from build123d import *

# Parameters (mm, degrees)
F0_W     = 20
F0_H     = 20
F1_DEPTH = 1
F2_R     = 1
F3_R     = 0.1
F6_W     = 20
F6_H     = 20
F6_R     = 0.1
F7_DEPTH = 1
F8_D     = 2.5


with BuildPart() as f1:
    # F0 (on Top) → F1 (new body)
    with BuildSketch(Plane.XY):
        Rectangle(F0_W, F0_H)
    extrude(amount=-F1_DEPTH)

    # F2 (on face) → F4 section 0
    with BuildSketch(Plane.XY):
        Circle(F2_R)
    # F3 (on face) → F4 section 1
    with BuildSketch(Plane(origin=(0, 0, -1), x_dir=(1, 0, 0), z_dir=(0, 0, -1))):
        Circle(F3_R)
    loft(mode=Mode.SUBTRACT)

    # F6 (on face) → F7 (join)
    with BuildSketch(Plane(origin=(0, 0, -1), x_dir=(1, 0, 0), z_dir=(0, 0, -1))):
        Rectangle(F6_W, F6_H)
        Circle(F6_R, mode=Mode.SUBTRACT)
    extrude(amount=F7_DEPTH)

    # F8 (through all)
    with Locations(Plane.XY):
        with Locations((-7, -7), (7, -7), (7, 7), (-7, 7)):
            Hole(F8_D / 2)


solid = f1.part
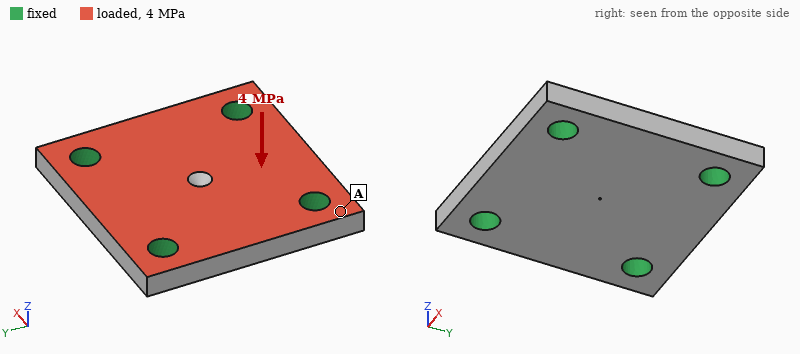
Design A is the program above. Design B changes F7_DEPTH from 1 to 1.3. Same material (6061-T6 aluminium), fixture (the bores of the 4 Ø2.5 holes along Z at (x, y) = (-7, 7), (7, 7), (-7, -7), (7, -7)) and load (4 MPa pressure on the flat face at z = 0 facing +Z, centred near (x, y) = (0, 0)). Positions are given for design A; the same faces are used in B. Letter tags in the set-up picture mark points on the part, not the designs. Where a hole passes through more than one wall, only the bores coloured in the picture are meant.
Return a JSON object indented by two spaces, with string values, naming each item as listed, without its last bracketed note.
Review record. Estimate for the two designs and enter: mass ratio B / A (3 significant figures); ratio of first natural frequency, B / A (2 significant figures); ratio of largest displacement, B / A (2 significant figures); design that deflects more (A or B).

{
  "mass ratio B / A": "1.15",
  "ratio of first natural frequency, B / A": "1.1",
  "ratio of largest displacement, B / A": "0.71",
  "design that deflects more": "A"
}
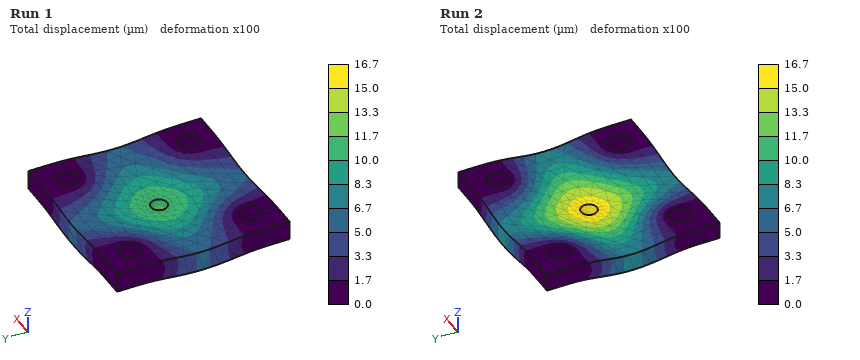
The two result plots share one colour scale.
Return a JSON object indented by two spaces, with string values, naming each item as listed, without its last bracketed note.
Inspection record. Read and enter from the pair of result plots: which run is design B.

{
  "which run is design B": "Run 1"
}
